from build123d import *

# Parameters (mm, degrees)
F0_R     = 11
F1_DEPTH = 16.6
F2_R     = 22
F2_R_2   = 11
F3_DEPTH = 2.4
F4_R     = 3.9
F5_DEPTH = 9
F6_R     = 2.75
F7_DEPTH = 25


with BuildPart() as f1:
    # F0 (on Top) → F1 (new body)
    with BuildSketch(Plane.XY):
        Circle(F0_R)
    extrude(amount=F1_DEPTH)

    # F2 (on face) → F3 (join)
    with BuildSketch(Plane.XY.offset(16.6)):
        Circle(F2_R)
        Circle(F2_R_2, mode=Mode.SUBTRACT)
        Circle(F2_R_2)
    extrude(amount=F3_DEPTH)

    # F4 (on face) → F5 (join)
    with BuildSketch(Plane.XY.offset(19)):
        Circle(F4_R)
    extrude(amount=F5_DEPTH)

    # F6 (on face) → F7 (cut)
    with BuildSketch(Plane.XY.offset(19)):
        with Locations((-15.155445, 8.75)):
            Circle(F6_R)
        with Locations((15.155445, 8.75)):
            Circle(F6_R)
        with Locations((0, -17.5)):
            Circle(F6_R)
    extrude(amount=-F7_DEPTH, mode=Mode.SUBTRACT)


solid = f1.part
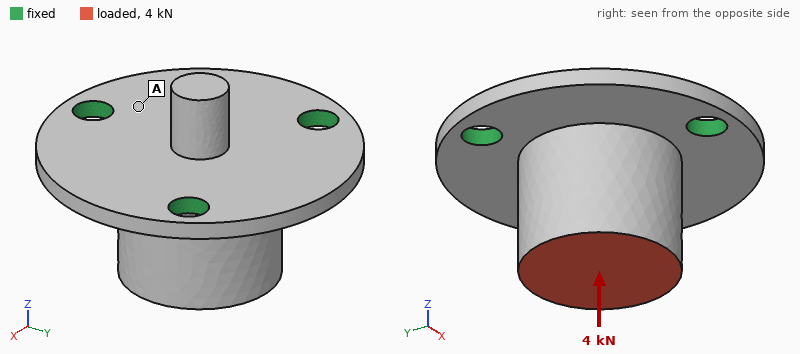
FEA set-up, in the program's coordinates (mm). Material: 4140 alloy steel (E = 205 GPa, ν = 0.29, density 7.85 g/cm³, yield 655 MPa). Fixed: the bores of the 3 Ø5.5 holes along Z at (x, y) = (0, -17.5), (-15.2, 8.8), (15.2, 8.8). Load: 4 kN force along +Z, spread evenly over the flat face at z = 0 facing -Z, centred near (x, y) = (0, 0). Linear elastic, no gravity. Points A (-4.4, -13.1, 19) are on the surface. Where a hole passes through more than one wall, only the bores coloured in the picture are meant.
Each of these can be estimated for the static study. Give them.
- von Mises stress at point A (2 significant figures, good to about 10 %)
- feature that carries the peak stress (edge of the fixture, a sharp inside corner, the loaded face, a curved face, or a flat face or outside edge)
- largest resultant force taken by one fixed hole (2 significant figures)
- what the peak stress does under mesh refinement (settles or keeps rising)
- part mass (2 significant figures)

57 MPa
edge of the fixture
1.4 kN
keeps rising
80 g
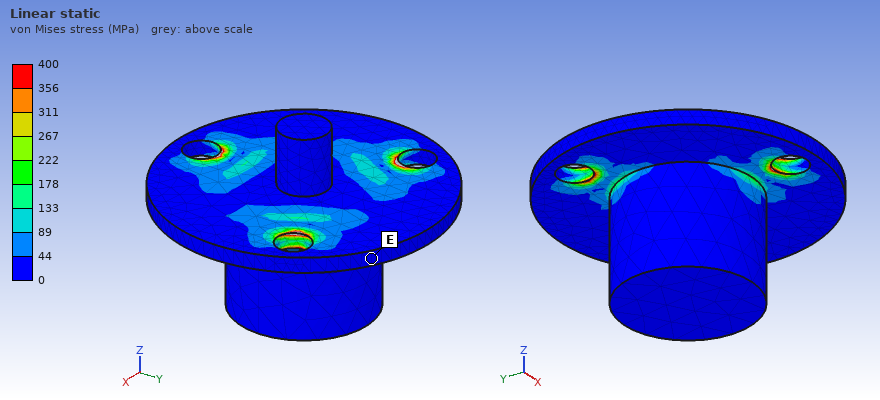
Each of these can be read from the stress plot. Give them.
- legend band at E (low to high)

0 to 44 MPa
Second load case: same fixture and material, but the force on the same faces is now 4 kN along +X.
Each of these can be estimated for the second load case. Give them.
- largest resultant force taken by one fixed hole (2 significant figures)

3.3 kN
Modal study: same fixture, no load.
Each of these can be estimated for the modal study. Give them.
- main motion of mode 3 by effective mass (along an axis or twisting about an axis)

along Z
